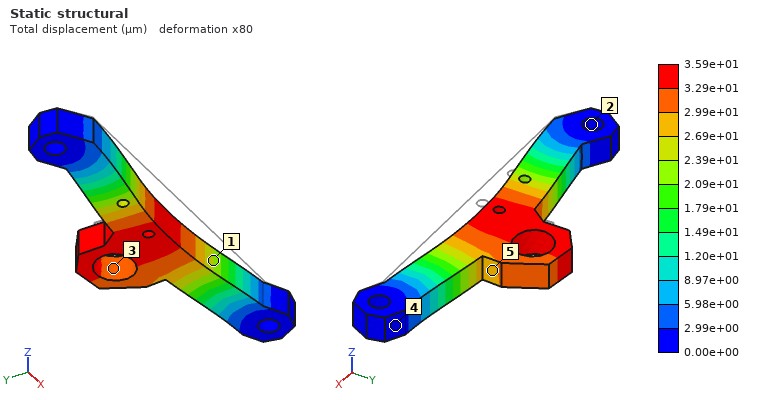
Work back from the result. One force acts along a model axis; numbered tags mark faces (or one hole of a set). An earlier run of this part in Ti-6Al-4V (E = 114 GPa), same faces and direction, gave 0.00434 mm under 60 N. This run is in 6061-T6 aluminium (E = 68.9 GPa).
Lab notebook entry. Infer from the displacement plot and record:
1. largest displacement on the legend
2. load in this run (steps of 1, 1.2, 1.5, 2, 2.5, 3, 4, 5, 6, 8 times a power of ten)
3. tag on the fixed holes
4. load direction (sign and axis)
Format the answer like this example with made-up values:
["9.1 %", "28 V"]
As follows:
["3.59e+01 µm", "300 N", "2", "+Y"]
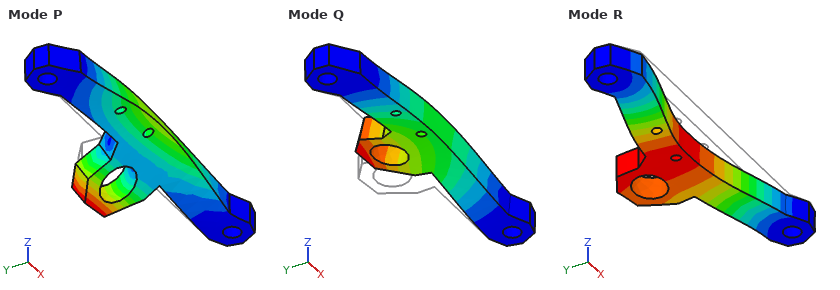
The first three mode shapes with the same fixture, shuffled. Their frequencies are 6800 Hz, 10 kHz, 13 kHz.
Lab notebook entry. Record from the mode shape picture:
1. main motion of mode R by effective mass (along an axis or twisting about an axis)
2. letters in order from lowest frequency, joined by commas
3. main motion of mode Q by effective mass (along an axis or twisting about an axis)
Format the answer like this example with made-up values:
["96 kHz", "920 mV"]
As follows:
["along Y", "Q, R, P", "along Z"]
